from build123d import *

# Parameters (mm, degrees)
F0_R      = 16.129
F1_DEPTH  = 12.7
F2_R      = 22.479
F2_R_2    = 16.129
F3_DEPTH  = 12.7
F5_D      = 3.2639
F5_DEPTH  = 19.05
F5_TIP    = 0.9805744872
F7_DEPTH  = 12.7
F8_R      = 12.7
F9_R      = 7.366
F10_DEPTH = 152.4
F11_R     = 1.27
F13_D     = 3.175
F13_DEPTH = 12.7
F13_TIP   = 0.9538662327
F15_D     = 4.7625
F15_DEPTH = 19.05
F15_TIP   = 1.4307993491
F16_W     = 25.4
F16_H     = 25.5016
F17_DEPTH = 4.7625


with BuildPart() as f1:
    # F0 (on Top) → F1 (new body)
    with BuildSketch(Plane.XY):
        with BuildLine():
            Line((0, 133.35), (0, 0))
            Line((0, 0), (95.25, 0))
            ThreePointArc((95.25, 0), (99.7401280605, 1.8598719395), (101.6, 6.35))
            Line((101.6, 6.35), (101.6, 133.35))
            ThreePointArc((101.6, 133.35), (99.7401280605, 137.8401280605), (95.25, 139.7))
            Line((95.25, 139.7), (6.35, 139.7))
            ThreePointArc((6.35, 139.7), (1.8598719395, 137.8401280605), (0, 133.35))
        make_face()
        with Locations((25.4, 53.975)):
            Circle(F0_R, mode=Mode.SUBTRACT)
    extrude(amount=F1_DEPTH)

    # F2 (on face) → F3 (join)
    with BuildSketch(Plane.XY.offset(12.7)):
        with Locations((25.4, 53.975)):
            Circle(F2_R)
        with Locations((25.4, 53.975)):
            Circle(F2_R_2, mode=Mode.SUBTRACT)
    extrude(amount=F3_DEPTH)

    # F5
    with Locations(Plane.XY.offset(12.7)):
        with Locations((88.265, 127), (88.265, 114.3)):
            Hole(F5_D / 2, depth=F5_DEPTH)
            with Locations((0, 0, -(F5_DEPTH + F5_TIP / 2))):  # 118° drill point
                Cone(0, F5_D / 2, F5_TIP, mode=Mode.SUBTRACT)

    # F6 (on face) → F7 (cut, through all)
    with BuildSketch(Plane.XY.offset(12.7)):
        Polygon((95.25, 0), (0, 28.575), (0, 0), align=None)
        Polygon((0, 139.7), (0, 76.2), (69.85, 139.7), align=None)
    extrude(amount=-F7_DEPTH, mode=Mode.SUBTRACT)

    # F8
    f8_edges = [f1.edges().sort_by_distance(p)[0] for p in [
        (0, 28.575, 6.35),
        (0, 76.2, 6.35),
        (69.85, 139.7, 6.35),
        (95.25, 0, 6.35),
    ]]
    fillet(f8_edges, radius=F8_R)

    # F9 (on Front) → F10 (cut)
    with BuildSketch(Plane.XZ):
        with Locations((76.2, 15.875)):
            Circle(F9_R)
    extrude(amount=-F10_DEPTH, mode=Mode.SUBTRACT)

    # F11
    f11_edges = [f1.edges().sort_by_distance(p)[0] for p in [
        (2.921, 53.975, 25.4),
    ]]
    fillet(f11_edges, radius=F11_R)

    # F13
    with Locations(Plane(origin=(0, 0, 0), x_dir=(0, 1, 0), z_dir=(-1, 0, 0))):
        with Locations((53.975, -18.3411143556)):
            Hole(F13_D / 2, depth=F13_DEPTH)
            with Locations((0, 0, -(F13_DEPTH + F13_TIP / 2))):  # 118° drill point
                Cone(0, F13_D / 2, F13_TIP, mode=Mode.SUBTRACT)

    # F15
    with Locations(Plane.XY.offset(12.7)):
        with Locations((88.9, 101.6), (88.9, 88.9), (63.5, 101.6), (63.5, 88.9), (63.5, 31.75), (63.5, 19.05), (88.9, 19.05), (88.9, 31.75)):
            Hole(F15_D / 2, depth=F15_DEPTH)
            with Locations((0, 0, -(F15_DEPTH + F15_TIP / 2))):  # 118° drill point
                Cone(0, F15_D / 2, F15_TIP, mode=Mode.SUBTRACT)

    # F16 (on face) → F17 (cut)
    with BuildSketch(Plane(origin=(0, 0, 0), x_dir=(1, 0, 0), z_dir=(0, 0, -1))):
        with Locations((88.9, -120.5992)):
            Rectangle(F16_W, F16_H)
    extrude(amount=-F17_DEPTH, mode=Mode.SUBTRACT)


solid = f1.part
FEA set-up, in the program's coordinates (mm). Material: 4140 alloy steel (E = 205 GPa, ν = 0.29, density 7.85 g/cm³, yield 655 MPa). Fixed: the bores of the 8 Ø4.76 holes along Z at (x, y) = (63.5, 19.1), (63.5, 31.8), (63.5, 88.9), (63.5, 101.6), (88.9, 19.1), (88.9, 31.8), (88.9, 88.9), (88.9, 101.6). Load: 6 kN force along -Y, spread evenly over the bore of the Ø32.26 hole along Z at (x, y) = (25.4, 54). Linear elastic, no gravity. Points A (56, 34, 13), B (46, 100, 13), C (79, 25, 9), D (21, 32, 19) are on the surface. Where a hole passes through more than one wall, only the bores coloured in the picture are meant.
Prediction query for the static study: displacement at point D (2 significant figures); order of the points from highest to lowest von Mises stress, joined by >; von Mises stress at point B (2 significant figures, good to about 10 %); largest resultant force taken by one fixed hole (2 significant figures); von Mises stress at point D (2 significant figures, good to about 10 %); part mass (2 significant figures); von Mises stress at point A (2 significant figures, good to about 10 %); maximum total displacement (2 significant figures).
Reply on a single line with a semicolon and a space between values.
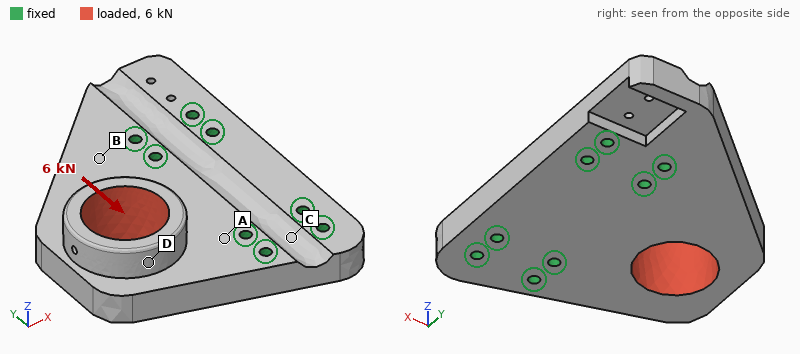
8.3 µm; A > D > B > C; 5.8 MPa; 2.4 kN; 9.1 MPa; 960 g; 12 MPa; 11 µm
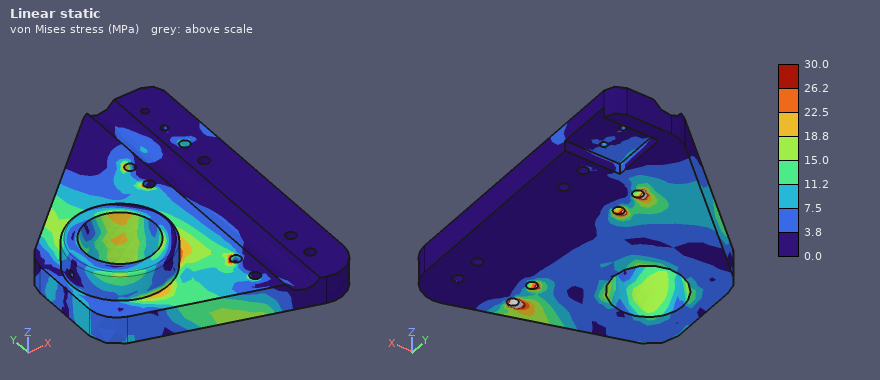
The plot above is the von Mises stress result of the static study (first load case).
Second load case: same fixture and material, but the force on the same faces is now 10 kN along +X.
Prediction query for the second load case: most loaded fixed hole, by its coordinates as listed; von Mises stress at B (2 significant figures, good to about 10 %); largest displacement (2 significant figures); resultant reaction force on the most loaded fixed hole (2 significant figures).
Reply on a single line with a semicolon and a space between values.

(63.5, 31.8); 23 MPa; 41 µm; 3.2 kN
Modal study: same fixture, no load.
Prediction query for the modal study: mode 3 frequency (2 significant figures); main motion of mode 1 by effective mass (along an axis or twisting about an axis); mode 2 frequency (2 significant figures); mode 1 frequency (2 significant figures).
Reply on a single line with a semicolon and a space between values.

6500 Hz; along Z; 6100 Hz; 2700 Hz
